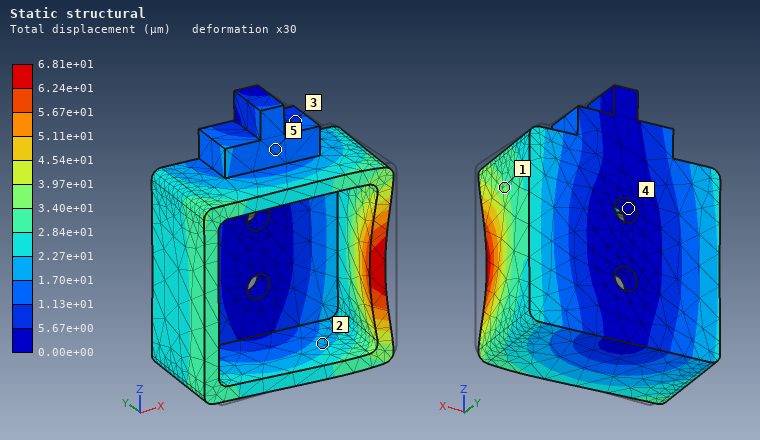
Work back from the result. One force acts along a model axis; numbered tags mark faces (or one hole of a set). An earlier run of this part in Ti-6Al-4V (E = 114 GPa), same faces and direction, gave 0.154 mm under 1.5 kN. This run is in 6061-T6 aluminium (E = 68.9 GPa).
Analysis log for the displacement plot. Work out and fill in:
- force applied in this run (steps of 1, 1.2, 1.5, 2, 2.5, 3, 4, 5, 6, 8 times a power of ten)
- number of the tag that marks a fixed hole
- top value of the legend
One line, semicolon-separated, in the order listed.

400 N; 4; 6.81e+01 µm
